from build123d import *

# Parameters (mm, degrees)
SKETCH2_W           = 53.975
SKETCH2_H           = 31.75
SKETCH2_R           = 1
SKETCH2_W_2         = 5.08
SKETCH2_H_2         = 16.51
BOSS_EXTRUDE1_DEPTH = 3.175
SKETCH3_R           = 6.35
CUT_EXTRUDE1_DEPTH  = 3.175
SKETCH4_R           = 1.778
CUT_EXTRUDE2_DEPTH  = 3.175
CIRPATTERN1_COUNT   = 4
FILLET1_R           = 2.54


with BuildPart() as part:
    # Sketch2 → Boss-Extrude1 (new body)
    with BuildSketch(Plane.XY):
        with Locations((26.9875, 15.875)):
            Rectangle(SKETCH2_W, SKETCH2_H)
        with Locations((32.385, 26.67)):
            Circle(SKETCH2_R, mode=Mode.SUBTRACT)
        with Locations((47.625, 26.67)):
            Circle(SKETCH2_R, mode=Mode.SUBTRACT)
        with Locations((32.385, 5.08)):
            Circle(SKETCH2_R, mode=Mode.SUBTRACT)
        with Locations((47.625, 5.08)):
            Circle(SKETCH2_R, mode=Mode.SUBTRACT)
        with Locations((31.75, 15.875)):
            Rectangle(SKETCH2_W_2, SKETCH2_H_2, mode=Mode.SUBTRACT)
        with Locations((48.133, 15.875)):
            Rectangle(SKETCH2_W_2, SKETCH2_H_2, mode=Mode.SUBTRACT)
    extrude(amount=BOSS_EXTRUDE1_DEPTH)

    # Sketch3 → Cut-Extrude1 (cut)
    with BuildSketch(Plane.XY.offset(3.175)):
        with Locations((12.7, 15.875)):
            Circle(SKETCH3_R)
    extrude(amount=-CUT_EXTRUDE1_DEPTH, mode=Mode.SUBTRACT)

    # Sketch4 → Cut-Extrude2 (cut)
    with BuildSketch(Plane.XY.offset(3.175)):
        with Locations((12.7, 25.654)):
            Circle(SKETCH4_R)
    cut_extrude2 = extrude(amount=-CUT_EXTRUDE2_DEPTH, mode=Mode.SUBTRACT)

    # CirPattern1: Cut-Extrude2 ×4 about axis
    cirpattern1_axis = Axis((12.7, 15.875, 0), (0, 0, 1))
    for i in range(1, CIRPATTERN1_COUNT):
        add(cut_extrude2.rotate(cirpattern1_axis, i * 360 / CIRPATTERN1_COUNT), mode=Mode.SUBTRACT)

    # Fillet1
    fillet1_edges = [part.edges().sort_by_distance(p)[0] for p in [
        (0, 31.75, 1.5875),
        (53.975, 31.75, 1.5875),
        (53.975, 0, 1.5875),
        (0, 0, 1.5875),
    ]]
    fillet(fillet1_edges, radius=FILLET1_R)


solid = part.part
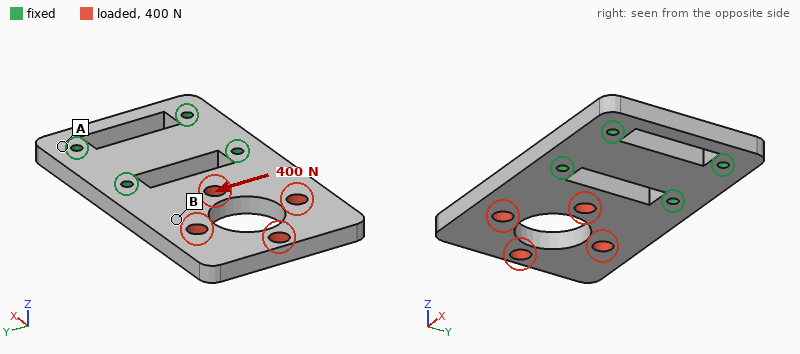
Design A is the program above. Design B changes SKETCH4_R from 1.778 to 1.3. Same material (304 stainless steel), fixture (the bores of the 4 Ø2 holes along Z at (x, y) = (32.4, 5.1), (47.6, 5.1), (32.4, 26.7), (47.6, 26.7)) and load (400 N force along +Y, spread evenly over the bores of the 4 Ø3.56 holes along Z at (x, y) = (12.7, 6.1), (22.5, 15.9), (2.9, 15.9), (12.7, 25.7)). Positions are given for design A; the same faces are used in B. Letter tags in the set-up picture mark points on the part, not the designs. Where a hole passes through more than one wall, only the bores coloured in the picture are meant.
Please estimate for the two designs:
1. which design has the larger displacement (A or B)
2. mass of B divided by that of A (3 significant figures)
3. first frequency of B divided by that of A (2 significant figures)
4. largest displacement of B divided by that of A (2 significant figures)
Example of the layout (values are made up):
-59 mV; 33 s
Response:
A; 1.01; 0.99; 0.89
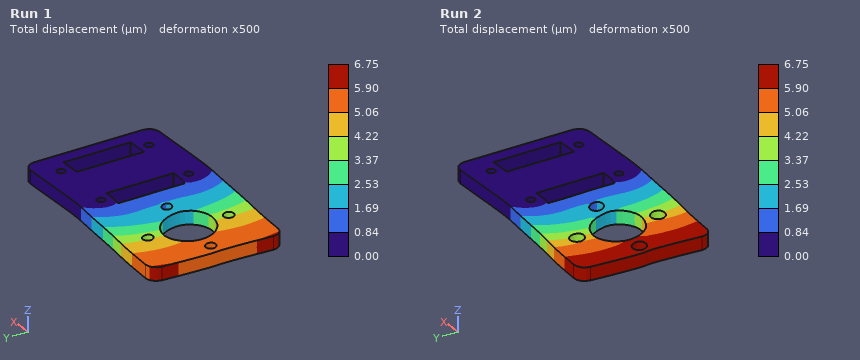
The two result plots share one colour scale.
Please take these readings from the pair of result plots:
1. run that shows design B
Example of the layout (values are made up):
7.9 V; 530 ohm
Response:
Run 1
